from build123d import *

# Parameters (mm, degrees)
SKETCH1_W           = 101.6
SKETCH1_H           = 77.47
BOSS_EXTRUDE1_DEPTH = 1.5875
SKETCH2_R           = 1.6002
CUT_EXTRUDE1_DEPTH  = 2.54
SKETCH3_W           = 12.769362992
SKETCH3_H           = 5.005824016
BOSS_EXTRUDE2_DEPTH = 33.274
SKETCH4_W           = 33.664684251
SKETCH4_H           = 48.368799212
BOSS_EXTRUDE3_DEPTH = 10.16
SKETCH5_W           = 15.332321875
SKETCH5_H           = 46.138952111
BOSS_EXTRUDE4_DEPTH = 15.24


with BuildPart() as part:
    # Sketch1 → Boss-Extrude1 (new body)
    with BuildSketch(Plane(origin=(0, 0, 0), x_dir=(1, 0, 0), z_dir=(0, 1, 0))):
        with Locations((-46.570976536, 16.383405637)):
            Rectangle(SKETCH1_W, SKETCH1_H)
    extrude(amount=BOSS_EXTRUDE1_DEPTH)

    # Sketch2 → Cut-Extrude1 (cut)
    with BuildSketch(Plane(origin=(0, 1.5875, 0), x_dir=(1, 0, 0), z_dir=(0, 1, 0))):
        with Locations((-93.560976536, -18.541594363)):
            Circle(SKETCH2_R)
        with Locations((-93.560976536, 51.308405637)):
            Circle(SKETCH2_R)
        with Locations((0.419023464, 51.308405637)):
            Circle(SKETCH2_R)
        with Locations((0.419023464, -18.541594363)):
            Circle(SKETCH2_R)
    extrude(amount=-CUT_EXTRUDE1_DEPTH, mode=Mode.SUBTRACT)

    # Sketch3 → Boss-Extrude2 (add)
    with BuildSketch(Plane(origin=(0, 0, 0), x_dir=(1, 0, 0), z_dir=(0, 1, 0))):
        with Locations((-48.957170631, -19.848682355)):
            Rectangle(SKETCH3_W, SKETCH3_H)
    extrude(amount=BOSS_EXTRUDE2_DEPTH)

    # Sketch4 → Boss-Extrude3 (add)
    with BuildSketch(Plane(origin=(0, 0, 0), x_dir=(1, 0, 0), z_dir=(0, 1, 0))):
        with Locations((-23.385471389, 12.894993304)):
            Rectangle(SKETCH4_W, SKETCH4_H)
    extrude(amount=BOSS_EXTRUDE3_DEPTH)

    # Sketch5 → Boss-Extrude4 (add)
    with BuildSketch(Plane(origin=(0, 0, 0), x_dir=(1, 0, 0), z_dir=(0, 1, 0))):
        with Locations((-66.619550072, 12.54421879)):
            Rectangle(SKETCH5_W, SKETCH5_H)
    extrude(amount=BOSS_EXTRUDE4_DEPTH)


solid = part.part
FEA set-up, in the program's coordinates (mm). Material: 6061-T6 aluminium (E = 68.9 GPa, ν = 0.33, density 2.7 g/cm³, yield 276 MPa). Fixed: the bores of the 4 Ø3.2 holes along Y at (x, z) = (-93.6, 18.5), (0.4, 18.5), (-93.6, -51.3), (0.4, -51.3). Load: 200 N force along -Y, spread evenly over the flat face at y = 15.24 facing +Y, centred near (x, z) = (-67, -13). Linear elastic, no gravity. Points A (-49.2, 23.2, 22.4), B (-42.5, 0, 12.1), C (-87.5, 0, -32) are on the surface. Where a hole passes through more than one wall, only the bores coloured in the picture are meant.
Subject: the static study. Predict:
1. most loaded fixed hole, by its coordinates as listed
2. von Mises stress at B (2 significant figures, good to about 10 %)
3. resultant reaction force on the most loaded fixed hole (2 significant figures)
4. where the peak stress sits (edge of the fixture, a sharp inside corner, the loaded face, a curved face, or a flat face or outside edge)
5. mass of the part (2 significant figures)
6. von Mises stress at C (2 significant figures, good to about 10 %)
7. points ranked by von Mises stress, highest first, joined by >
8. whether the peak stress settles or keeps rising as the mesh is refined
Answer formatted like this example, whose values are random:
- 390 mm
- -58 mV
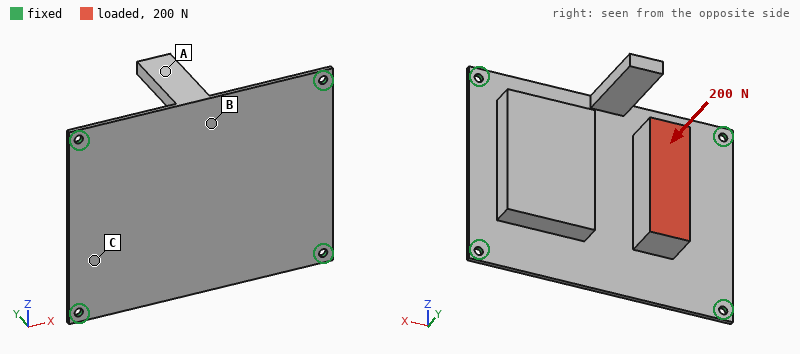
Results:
- (-93.6, 18.5)
- 40 MPa
- 92 N
- edge of the fixture
- 100 g
- 20 MPa
- B > C > A
- keeps rising
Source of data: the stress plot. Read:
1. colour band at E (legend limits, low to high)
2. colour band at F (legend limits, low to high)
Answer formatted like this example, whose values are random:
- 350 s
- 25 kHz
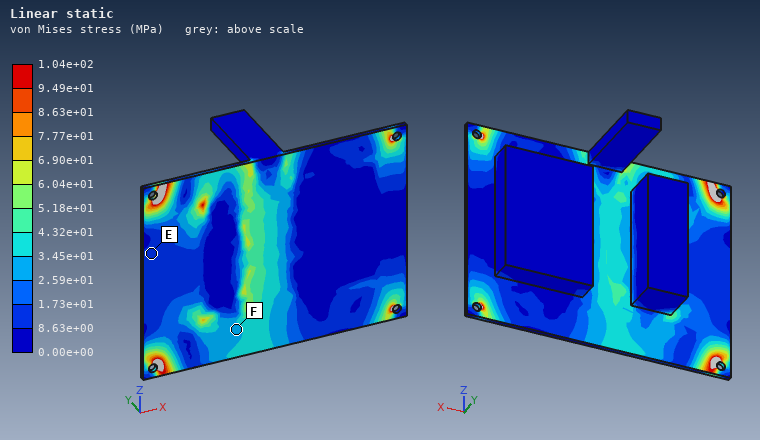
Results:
- 8.63e+00 to 1.73e+01 MPa
- 2.59e+01 to 3.45e+01 MPa
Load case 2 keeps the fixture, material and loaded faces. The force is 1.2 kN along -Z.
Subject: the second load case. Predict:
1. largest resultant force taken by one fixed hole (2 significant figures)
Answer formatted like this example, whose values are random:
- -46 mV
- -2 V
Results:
- 430 N
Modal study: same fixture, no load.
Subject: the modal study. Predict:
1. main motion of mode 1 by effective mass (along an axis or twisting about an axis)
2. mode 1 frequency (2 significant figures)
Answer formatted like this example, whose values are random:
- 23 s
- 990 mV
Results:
- along Y
- 460 Hz
